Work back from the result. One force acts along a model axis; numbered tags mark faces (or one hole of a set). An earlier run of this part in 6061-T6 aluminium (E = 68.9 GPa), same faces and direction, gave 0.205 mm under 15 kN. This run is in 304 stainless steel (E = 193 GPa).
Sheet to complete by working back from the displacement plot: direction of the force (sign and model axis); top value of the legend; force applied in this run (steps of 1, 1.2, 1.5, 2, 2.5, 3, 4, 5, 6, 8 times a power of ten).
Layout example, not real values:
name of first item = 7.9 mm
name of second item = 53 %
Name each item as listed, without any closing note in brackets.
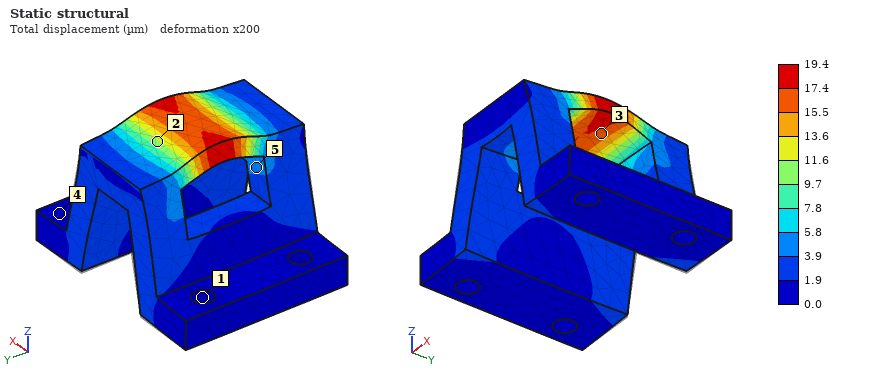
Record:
direction of the force = +Z
top value of the legend = 19.4 µm
force applied in this run = 4 kN
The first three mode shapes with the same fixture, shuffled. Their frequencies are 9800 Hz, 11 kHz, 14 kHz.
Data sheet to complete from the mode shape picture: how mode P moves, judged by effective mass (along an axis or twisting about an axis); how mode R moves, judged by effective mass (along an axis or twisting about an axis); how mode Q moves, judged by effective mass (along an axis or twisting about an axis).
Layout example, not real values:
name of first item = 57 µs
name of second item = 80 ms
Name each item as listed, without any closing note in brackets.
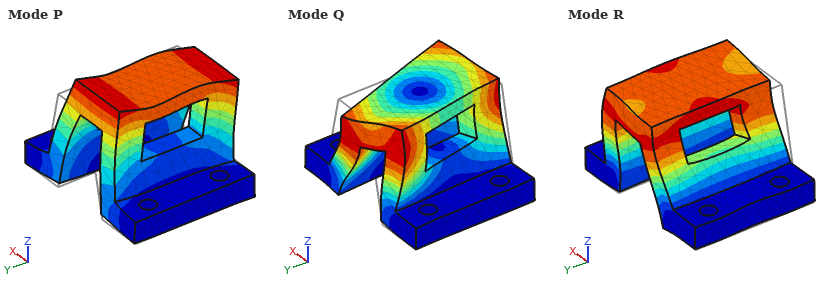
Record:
how mode P moves, judged by effective mass = along Y
how mode R moves, judged by effective mass = along X
how mode Q moves, judged by effective mass = twisting about Z
